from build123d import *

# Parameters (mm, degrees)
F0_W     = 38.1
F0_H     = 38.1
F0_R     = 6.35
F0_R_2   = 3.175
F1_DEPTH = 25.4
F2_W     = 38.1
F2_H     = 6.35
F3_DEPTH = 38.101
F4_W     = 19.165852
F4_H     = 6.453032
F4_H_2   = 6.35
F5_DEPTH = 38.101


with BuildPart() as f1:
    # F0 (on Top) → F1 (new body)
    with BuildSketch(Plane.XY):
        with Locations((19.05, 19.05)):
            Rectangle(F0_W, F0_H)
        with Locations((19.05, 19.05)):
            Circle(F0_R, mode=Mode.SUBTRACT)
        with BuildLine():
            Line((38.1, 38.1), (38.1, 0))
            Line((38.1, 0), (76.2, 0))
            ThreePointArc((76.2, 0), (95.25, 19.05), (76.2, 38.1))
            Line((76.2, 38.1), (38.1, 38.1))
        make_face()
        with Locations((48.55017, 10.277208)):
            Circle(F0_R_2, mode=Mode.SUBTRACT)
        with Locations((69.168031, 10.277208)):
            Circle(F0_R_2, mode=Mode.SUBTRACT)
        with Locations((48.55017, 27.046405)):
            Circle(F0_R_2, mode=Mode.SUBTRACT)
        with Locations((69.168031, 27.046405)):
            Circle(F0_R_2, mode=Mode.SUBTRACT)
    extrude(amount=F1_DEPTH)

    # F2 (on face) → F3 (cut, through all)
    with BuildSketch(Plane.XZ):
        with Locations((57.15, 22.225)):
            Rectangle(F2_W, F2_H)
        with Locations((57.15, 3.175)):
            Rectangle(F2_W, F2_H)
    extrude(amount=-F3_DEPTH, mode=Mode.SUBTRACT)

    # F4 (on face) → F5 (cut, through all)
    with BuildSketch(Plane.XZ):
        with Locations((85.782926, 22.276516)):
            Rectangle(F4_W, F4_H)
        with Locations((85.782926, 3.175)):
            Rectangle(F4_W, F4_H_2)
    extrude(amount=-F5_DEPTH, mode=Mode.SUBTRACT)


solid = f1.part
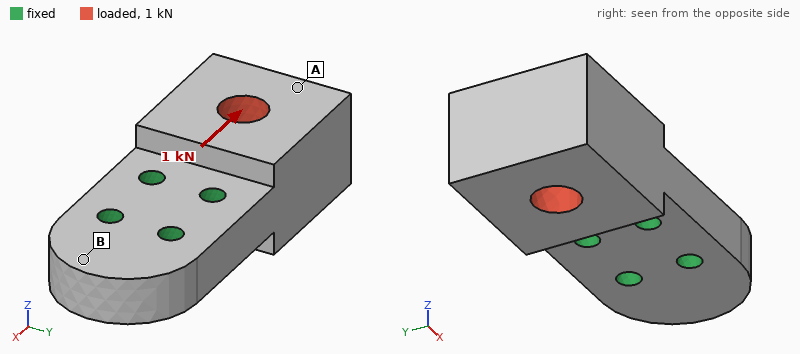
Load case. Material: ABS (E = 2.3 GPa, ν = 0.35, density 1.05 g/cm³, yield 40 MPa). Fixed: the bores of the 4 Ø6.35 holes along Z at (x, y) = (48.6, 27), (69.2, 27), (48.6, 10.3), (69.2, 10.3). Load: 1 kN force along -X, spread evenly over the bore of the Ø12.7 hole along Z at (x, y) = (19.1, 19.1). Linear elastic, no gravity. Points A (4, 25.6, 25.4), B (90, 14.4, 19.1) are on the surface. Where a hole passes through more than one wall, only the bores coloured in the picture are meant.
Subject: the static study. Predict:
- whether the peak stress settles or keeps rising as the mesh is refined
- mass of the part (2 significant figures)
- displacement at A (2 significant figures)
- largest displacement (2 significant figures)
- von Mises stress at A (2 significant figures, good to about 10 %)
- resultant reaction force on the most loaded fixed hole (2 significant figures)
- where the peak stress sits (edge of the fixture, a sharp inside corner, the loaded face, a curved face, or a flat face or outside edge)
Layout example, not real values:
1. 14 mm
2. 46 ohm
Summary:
1. keeps rising
2. 61 g
3. 26 µm
4. 31 µm
5. 0.72 MPa
6. 470 N
7. edge of the fixture
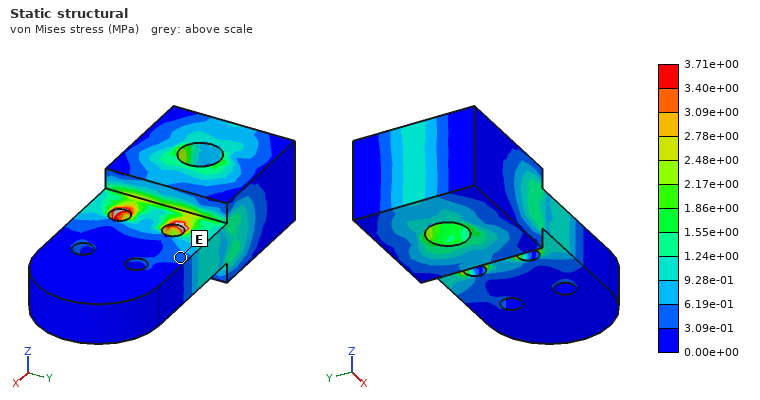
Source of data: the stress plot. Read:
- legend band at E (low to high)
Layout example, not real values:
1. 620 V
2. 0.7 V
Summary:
1. 3.09e-01 to 6.19e-01 MPa
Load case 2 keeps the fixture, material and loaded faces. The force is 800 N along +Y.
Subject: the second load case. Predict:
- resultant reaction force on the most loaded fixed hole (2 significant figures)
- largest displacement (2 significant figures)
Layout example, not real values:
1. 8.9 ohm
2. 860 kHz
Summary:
1. 940 N
2. 0.19 mm
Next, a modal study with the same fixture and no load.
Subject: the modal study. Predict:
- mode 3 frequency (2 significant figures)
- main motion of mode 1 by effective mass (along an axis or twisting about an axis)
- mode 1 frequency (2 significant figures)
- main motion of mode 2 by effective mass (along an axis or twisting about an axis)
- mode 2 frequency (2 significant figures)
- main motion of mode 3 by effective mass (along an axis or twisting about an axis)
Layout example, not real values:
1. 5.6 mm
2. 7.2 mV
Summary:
1. 2700 Hz
2. along Z
3. 1000 Hz
4. along Y
5. 2000 Hz
6. twisting about X
